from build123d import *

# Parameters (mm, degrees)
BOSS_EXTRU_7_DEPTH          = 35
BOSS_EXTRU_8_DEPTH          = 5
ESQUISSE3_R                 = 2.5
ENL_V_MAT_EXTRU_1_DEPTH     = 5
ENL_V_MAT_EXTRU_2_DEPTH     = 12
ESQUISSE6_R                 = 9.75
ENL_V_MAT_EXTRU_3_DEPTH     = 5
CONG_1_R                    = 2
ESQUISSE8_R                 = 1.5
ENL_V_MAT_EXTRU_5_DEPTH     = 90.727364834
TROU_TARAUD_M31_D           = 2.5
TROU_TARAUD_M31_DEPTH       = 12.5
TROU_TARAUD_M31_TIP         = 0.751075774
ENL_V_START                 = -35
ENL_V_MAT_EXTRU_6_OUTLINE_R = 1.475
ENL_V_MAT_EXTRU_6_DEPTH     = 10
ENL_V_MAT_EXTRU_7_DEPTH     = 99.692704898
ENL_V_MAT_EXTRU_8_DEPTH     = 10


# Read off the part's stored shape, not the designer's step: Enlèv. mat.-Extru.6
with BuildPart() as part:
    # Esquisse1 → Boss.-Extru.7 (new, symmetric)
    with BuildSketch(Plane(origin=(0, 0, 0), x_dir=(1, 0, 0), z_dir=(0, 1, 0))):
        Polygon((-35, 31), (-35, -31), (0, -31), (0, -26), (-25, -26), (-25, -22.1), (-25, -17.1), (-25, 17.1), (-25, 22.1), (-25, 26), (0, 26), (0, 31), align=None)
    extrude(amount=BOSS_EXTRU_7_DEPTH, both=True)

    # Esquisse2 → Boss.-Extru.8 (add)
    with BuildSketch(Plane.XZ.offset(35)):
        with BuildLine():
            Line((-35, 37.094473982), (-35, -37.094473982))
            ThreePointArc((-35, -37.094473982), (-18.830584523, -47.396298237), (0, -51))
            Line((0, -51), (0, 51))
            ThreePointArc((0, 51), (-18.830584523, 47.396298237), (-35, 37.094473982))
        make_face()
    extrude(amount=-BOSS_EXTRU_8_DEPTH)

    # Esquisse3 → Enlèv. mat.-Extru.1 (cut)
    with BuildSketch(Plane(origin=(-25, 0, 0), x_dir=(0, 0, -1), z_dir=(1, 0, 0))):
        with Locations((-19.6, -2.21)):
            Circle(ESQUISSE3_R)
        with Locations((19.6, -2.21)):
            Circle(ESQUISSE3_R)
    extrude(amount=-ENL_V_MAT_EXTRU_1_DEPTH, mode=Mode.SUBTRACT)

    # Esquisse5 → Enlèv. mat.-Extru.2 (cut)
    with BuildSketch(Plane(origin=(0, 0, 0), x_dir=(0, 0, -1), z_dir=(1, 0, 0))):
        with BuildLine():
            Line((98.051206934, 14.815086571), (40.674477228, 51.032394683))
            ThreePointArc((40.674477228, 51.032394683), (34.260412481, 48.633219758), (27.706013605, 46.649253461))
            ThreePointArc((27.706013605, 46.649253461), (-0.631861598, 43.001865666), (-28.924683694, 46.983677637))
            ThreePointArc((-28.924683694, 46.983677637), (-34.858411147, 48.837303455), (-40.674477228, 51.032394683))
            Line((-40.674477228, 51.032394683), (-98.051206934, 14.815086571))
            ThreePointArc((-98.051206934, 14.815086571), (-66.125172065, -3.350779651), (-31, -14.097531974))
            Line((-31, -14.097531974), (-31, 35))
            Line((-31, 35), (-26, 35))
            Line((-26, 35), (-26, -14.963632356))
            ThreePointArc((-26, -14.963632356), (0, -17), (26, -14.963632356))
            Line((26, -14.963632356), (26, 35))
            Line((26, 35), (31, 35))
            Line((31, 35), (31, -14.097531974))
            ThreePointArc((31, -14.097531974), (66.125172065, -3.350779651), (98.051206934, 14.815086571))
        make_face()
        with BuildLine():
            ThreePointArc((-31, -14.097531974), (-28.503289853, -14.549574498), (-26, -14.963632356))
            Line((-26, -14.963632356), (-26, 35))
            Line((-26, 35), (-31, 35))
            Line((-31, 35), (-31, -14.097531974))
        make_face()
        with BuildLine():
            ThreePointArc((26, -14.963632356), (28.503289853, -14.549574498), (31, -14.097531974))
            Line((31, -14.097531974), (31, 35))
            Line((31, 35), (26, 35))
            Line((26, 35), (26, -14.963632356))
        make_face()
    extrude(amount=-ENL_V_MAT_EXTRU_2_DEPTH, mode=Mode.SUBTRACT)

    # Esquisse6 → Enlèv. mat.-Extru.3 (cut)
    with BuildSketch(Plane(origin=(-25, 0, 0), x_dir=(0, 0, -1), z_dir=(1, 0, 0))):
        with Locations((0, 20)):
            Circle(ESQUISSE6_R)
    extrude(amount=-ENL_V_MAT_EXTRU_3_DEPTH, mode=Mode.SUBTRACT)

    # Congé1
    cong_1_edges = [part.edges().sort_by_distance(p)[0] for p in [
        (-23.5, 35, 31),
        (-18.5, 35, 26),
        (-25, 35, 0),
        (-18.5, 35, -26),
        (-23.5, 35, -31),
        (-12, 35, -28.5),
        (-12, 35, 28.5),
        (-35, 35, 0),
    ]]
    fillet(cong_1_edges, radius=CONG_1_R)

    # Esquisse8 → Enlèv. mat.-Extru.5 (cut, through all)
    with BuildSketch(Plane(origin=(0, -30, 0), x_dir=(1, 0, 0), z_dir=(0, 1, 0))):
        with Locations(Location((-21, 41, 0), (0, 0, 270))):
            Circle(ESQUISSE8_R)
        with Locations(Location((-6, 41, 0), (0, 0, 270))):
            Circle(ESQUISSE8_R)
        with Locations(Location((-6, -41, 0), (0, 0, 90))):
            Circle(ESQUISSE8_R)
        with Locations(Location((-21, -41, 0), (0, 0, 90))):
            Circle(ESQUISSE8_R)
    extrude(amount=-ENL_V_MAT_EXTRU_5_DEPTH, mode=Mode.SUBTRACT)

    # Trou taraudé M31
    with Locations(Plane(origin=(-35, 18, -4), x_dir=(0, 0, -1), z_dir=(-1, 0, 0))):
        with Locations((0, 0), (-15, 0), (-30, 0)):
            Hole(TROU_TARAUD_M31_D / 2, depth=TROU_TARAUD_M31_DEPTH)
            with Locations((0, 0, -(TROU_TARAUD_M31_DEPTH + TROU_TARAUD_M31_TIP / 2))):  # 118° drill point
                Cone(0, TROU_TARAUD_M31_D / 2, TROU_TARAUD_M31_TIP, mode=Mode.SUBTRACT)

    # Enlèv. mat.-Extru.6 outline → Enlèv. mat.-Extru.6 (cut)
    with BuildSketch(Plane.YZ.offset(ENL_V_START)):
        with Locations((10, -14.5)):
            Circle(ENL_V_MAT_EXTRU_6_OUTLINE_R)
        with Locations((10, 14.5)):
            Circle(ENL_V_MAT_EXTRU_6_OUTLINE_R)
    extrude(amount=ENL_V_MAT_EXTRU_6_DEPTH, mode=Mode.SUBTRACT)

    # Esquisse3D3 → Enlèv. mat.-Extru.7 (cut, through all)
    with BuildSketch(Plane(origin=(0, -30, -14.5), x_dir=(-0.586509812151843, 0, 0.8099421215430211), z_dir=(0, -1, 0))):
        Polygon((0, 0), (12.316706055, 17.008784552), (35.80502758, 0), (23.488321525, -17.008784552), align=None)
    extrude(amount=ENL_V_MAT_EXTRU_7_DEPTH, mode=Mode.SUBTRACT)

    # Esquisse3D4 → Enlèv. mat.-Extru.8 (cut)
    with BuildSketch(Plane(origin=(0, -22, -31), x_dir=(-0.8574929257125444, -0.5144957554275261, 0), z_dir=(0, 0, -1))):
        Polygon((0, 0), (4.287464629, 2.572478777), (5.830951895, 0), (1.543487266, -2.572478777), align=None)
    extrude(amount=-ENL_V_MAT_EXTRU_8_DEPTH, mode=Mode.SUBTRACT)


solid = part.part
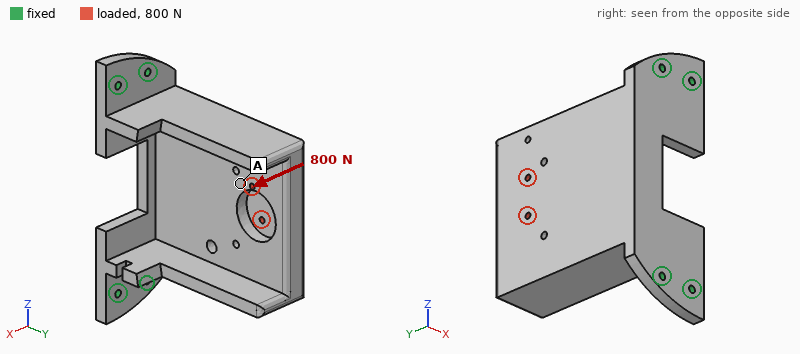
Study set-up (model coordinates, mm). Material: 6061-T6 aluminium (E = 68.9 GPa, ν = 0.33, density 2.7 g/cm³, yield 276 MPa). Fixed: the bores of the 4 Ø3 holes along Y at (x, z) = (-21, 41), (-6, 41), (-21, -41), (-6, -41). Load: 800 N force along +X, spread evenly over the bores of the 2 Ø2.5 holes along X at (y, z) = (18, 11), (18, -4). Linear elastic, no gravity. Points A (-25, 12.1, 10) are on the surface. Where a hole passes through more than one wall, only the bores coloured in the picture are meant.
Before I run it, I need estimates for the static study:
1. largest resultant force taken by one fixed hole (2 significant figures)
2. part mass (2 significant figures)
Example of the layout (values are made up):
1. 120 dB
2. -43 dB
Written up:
1. 1.2 kN
2. 170 g
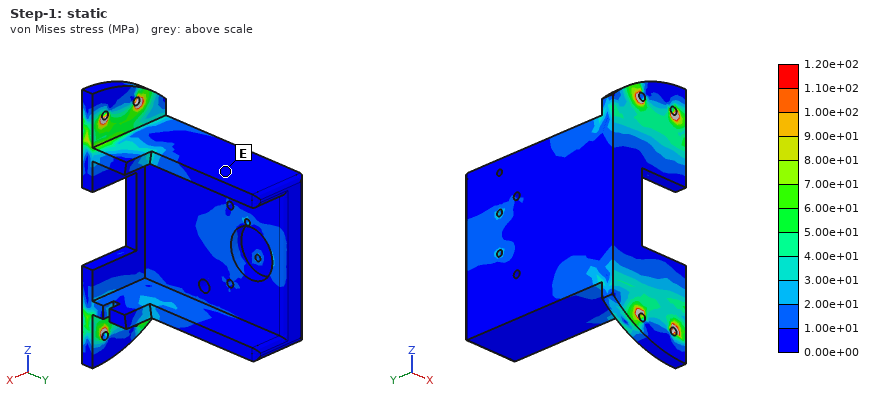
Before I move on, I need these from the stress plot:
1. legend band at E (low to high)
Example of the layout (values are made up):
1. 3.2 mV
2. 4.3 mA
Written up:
1. 0.00e+00 to 1.00e+01 MPa
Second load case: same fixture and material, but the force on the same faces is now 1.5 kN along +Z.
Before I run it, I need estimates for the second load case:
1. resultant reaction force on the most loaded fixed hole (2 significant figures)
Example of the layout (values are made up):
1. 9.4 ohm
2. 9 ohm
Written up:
1. 1.1 kN
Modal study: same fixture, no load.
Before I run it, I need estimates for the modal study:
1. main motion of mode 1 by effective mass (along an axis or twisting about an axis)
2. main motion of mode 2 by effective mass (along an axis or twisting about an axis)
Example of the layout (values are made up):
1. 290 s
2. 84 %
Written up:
1. along X
2. along Z
